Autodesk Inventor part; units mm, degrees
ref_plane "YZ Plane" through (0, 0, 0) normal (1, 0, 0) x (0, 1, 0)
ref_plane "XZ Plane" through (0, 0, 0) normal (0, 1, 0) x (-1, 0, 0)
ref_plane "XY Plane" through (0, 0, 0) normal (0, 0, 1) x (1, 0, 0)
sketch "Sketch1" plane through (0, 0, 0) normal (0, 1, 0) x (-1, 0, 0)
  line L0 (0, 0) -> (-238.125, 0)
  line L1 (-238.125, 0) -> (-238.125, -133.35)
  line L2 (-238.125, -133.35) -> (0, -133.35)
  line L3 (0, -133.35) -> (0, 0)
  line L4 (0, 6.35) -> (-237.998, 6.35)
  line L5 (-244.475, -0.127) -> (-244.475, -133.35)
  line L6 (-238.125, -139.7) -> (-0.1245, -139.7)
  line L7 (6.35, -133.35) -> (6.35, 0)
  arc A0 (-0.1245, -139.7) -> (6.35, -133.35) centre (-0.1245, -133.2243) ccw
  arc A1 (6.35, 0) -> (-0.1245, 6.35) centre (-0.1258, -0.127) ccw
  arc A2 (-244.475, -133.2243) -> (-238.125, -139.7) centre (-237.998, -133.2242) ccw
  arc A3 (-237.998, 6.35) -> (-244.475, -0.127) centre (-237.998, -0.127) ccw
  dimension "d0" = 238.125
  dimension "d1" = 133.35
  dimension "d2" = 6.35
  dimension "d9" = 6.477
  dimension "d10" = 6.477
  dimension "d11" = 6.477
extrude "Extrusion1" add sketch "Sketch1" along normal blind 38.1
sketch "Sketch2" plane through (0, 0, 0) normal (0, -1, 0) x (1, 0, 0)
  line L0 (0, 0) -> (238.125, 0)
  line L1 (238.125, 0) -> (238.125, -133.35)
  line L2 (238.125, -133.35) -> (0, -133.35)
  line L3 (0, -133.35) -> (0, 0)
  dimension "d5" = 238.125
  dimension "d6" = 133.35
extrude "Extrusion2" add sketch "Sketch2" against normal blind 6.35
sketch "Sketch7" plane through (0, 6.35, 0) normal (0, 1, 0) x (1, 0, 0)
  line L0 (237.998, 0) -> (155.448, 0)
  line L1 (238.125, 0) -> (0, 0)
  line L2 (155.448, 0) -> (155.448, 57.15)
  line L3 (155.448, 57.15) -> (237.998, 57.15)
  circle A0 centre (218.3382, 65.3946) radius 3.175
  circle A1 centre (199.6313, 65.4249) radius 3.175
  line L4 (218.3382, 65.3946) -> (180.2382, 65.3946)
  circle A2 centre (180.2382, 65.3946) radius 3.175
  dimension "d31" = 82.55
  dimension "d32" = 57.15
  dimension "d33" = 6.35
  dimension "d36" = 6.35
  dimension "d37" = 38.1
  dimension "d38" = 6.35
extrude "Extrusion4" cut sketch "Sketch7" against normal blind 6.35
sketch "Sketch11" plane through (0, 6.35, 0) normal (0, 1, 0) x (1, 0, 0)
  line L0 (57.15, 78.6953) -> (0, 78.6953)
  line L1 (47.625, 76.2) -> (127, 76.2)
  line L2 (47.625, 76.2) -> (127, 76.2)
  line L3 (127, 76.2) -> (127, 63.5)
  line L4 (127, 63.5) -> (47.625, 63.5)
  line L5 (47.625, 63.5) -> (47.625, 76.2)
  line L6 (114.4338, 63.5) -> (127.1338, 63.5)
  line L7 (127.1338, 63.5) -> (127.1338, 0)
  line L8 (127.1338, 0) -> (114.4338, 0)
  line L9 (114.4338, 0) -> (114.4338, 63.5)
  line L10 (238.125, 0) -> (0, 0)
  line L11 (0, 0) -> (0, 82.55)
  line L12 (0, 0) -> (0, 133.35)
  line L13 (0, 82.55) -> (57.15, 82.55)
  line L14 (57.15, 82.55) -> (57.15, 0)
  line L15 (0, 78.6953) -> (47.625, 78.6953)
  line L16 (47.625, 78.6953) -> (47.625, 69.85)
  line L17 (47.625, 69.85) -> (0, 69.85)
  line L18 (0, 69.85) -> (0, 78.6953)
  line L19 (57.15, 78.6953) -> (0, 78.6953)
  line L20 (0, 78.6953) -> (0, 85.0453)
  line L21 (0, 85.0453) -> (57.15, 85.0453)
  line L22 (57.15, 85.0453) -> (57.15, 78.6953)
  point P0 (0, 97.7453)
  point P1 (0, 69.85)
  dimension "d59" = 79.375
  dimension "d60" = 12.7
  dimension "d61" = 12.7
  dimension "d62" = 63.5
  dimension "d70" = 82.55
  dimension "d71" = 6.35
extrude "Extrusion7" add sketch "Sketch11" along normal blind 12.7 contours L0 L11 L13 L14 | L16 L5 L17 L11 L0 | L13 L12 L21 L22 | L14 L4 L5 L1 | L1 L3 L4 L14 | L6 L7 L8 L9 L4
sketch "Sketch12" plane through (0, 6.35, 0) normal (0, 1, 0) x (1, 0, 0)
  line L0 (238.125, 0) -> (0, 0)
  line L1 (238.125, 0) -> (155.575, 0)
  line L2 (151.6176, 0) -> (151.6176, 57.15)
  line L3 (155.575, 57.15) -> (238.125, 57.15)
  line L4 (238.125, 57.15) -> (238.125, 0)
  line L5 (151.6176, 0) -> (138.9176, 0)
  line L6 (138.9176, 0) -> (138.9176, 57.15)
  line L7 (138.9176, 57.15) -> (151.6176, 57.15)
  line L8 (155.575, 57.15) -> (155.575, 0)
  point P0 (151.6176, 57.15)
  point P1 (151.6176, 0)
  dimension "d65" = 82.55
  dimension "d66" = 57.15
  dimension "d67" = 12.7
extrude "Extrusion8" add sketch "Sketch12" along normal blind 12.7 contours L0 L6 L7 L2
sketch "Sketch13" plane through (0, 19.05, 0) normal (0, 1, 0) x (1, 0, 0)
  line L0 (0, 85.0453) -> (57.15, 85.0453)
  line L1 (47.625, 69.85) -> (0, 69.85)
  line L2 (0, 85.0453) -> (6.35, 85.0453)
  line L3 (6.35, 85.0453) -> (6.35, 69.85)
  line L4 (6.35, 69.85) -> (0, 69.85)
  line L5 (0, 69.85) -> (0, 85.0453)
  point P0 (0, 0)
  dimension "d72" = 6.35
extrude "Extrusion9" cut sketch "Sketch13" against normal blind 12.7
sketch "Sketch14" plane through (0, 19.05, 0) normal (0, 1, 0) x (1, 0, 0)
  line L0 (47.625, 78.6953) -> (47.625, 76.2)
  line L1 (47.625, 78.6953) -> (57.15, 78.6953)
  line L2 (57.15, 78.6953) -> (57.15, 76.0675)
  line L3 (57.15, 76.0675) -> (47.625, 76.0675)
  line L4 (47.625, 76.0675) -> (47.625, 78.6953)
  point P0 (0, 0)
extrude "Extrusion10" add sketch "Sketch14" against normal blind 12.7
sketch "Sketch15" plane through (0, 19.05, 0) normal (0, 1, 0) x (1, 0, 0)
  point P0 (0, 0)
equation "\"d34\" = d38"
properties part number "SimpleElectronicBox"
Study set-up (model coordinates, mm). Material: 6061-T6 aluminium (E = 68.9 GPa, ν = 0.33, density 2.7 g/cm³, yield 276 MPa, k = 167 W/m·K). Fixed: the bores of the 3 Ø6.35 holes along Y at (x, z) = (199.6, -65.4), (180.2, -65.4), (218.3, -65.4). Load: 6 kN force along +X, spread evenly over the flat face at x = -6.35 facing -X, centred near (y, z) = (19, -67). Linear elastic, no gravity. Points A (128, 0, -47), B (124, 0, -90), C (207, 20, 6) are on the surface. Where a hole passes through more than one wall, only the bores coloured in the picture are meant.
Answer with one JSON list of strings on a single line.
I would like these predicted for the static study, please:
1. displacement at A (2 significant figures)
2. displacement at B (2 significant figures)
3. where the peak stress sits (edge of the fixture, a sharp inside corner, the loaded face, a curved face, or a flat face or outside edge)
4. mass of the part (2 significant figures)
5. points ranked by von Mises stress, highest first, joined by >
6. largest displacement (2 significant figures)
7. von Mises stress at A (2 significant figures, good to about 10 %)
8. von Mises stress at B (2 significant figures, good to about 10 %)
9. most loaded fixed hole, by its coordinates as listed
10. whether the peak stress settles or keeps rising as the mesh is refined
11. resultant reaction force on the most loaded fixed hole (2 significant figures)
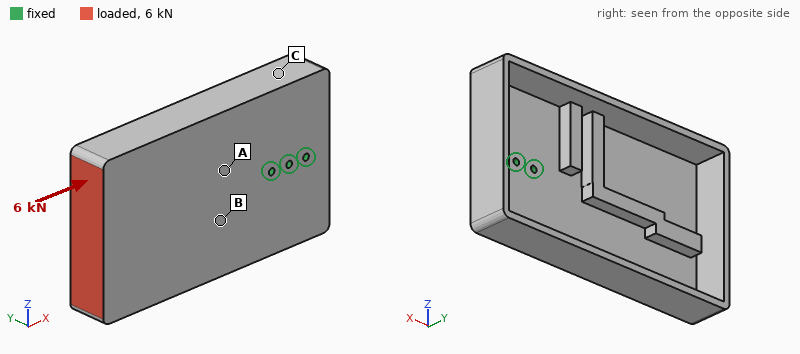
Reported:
["0.25 mm", "0.25 mm", "edge of the fixture", "1.2 kg", "B > A > C", "1.1 mm", "15 MPa", "21 MPa", "(180.2, -65.4)", "keeps rising", "3.6 kN"]
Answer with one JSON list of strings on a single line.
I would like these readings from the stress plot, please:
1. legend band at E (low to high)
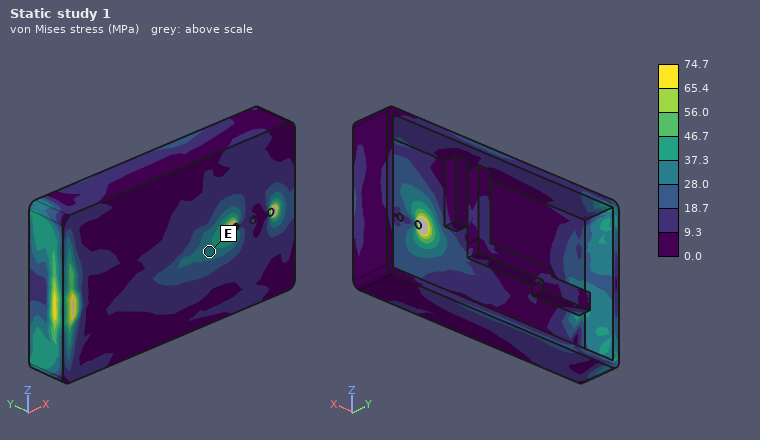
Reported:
["28.0 to 37.3 MPa"]
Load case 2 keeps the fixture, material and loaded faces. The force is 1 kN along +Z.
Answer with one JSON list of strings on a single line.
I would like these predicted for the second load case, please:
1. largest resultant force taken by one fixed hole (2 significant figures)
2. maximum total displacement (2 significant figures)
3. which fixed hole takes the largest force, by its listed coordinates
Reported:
["5.3 kN", "0.40 mm", "(180.2, -65.4)"]
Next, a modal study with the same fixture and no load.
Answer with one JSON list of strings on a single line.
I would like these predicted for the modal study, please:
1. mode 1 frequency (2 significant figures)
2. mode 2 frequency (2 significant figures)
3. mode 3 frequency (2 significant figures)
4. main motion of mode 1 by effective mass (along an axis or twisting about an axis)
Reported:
["190 Hz", "290 Hz", "720 Hz", "along Y"]
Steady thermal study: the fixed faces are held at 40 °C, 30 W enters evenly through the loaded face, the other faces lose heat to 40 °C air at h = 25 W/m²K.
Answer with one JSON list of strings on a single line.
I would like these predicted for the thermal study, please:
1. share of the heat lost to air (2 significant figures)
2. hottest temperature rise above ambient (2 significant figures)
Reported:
["67 %", "18 K"]
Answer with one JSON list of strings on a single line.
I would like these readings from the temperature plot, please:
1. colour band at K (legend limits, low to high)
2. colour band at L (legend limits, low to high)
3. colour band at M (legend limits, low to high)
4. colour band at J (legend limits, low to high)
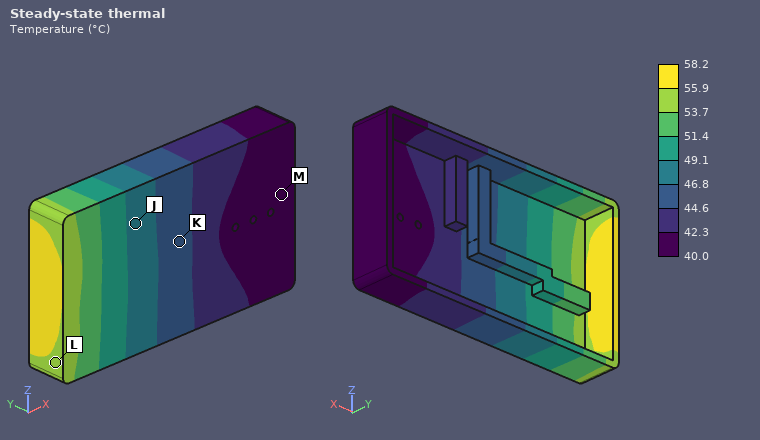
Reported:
["44.6 to 46.8 °C", "53.7 to 55.9 °C", "40.0 to 42.3 °C", "46.8 to 49.1 °C"]
